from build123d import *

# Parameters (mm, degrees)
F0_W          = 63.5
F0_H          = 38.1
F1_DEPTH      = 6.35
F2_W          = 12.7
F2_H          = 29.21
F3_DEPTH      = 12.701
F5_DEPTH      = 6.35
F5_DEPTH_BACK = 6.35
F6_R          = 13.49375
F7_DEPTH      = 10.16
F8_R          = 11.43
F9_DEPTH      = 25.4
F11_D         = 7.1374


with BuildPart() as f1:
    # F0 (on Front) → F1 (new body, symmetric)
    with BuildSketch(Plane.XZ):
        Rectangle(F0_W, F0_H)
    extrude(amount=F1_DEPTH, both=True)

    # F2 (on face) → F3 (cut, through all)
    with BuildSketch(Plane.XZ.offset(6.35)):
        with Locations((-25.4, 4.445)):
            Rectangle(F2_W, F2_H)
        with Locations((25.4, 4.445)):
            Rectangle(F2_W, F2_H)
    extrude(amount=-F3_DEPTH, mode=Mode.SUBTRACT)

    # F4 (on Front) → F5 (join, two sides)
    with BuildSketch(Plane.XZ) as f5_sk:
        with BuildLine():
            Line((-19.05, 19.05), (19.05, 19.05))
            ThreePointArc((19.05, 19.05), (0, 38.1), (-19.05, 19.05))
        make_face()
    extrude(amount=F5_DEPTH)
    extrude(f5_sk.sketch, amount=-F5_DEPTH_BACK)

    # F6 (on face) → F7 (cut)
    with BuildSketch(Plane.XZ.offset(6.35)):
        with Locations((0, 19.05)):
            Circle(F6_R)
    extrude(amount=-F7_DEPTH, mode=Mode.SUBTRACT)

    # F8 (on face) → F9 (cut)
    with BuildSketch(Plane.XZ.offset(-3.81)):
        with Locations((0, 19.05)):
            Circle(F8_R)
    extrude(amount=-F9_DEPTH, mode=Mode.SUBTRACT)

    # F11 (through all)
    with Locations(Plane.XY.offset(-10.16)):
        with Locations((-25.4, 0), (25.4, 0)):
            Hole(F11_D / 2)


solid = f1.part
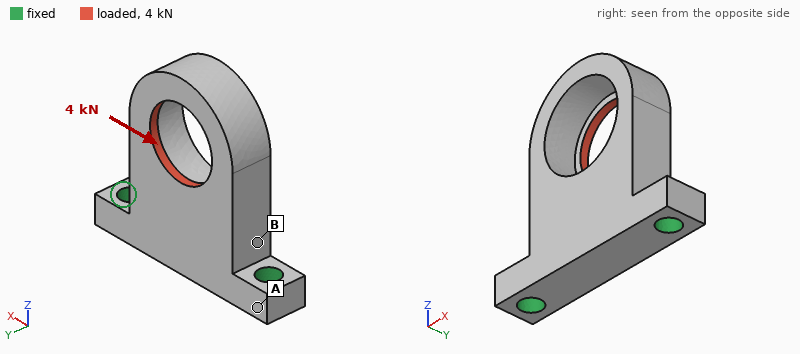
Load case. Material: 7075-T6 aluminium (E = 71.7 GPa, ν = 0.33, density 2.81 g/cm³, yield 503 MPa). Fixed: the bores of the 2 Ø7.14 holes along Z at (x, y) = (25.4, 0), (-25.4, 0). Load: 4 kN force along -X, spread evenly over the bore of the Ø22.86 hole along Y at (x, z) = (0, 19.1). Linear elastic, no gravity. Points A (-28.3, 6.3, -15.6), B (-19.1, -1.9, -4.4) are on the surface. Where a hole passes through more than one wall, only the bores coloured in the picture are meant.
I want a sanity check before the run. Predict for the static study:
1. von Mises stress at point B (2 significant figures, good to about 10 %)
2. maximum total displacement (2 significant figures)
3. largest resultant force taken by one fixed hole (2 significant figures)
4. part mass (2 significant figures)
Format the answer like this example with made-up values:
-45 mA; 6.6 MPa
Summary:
53 MPa; 0.13 mm; 3.9 kN; 59 g
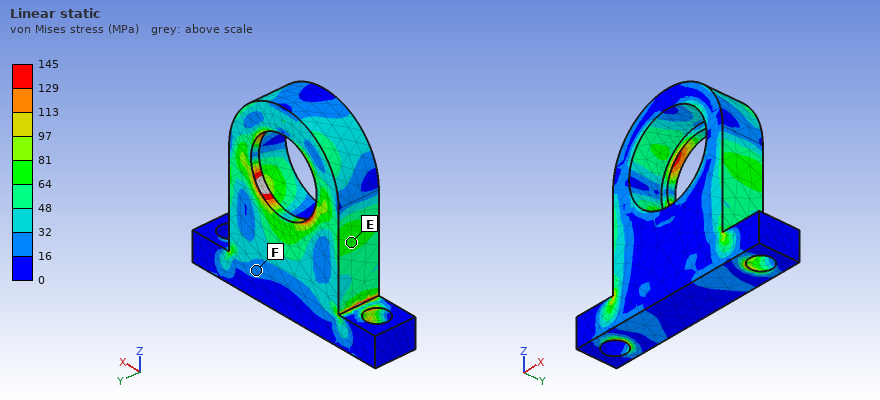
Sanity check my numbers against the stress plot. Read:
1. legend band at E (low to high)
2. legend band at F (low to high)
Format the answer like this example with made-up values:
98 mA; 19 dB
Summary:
64 to 81 MPa; 16 to 32 MPa
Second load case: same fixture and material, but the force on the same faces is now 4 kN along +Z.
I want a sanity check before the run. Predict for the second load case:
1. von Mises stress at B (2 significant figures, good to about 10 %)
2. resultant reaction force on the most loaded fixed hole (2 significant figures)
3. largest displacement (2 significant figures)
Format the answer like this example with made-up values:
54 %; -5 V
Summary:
16 MPa; 2.1 kN; 0.16 mm
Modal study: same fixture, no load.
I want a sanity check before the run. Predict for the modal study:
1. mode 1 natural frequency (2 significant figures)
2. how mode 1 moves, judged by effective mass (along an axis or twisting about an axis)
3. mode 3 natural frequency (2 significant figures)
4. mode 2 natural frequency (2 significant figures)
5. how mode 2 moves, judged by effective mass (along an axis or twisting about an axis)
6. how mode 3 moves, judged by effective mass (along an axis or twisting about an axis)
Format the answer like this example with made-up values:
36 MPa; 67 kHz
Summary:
2800 Hz; along Y; 9000 Hz; 7000 Hz; along X; twisting about Z
